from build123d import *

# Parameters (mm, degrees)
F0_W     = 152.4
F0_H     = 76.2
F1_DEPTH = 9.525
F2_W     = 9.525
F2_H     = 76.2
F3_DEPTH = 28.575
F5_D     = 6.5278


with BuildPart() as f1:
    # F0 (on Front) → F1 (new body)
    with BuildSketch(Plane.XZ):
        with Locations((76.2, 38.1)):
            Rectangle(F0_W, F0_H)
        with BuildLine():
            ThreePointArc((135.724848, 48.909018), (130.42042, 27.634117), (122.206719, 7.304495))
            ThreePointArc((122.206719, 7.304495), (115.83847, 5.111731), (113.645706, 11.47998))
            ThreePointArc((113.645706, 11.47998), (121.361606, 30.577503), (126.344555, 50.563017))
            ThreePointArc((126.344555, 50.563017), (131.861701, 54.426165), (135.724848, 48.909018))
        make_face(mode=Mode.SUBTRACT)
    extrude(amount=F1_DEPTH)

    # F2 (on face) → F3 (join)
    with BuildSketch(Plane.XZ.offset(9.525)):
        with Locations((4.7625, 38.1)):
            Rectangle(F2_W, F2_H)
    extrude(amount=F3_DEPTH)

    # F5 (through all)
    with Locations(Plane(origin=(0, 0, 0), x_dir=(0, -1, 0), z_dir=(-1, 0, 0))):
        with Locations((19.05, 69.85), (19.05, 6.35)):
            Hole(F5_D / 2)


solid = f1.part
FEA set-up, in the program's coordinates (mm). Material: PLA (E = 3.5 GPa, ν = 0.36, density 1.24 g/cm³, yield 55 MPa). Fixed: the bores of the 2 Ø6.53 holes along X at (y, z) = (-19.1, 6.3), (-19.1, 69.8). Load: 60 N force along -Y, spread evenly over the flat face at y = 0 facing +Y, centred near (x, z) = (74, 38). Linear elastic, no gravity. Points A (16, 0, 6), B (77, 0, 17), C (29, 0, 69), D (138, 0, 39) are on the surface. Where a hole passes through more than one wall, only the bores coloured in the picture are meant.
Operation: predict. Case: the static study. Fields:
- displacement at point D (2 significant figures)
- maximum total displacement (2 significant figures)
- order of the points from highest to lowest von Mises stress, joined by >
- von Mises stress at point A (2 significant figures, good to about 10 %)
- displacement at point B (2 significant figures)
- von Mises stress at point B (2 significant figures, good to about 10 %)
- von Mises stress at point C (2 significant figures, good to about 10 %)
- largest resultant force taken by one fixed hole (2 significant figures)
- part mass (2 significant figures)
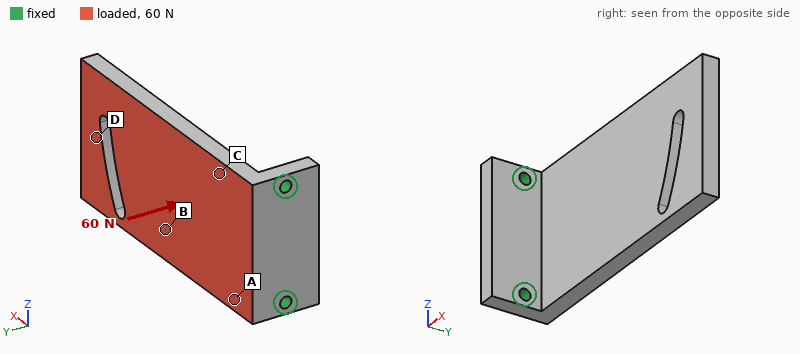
1.4 mm
1.6 mm
A > C > B > D
3.2 MPa
0.62 mm
0.90 MPa
2.6 MPa
32 N
160 g
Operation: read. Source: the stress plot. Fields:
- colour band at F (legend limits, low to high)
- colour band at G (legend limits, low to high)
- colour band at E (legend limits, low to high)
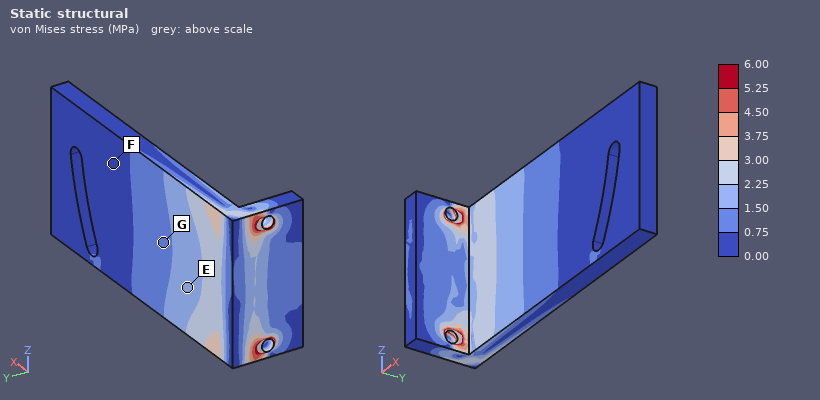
0.00 to 0.75 MPa
0.75 to 1.50 MPa
1.50 to 2.25 MPa
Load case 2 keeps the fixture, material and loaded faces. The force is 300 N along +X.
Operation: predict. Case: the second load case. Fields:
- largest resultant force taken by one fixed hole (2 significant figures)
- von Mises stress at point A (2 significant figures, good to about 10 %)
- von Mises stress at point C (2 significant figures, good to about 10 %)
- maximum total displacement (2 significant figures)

150 N
1.7 MPa
1.5 MPa
1.0 mm
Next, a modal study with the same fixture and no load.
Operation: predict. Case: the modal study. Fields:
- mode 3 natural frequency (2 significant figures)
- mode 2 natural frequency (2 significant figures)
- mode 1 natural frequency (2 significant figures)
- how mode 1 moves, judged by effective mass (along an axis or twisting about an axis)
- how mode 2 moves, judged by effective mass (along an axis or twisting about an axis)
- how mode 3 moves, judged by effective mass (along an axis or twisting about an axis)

530 Hz
430 Hz
110 Hz
along Y
along Z
along Z
